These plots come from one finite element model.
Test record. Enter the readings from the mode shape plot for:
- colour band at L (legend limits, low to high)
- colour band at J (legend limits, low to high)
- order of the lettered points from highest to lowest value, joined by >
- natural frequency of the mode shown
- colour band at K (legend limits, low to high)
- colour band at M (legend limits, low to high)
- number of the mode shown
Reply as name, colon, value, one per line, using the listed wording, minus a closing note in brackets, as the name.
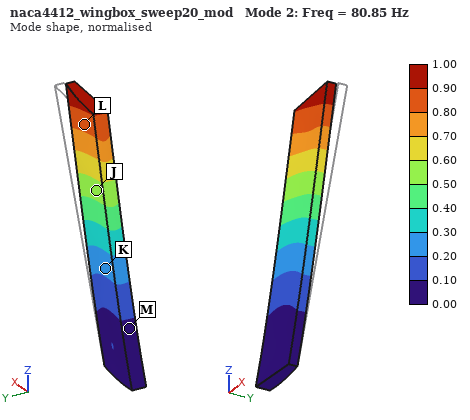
colour band at L: 0.80 to 0.90
colour band at J: 0.50 to 0.60
order of the lettered points from highest to lowest value, joined by >: L > J > K > M
natural frequency of the mode shown: 80.85 Hz
colour band at K: 0.20 to 0.30
colour band at M: 0.00 to 0.10
number of the mode shown: 2
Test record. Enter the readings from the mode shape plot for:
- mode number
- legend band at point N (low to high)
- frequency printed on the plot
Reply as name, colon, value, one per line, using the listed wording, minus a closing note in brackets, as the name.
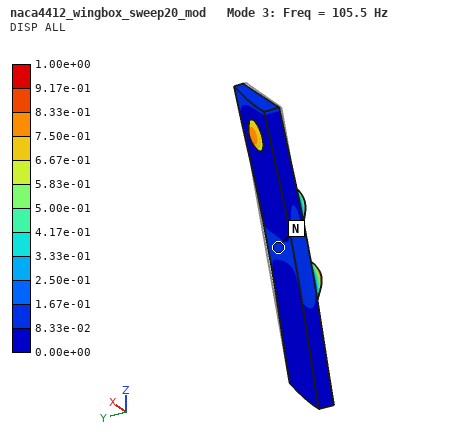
mode number: 3
legend band at point N: 8.33e-02 to 1.67e-01
frequency printed on the plot: 105.5 Hz
